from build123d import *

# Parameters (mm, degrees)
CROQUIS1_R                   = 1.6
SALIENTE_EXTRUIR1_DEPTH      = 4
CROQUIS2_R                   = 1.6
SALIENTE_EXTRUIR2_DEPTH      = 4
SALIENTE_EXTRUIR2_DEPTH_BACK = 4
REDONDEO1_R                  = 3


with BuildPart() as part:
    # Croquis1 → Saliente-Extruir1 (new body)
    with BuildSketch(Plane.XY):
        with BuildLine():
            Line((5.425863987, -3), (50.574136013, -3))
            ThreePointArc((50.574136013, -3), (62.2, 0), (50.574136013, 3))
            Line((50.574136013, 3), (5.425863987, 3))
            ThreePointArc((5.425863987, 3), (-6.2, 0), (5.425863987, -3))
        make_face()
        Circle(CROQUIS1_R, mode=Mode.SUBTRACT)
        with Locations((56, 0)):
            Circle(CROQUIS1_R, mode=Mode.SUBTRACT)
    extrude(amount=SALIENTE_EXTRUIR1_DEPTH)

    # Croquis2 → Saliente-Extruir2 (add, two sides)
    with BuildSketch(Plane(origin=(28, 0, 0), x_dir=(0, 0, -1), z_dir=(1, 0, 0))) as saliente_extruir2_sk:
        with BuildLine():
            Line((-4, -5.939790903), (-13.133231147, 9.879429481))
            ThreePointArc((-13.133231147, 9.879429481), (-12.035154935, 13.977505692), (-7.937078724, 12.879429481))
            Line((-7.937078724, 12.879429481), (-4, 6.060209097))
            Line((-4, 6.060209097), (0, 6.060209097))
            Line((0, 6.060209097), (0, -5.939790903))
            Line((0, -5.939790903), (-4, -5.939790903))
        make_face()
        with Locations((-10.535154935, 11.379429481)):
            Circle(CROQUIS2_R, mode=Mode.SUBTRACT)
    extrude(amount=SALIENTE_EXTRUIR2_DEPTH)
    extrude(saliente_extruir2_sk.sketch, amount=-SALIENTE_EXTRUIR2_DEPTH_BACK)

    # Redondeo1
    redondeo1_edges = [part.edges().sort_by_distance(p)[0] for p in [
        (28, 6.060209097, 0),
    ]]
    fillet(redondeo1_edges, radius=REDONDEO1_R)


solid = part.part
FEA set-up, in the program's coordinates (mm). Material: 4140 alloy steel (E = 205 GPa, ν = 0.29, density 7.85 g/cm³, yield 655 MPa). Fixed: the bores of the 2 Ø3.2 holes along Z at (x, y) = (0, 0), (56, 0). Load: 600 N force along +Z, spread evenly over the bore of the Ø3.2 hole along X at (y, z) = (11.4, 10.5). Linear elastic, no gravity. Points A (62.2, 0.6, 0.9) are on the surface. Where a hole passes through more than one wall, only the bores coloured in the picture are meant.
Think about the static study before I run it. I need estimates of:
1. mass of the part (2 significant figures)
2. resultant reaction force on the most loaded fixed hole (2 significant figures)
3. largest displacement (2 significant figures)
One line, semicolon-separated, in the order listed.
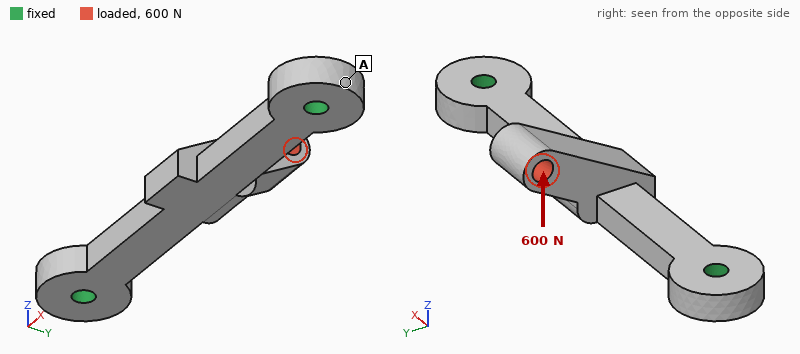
22 g; 310 N; 0.27 mm
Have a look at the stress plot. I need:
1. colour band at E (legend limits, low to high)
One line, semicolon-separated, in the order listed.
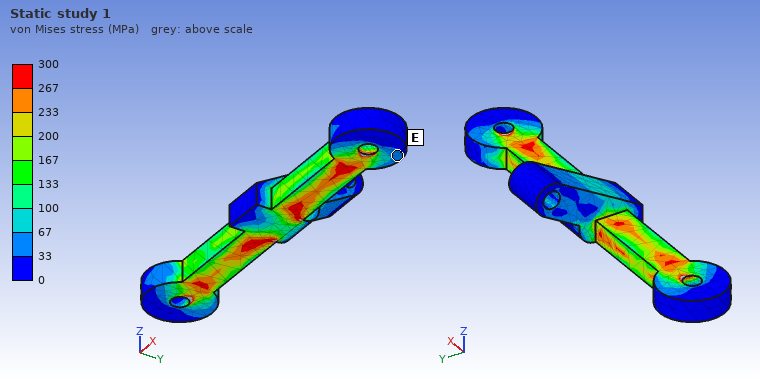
33 to 67 MPa
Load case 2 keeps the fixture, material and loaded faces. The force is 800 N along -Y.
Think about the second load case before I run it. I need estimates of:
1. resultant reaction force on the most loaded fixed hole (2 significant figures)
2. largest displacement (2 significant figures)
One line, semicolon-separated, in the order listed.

400 N; 0.25 mm
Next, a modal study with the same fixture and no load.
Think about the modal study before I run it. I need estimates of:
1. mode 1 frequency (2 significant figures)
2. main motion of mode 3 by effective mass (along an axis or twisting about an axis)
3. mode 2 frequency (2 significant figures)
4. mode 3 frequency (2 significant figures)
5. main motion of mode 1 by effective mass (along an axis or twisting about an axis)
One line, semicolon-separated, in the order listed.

4100 Hz; along Y; 5800 Hz; 8900 Hz; along Z
